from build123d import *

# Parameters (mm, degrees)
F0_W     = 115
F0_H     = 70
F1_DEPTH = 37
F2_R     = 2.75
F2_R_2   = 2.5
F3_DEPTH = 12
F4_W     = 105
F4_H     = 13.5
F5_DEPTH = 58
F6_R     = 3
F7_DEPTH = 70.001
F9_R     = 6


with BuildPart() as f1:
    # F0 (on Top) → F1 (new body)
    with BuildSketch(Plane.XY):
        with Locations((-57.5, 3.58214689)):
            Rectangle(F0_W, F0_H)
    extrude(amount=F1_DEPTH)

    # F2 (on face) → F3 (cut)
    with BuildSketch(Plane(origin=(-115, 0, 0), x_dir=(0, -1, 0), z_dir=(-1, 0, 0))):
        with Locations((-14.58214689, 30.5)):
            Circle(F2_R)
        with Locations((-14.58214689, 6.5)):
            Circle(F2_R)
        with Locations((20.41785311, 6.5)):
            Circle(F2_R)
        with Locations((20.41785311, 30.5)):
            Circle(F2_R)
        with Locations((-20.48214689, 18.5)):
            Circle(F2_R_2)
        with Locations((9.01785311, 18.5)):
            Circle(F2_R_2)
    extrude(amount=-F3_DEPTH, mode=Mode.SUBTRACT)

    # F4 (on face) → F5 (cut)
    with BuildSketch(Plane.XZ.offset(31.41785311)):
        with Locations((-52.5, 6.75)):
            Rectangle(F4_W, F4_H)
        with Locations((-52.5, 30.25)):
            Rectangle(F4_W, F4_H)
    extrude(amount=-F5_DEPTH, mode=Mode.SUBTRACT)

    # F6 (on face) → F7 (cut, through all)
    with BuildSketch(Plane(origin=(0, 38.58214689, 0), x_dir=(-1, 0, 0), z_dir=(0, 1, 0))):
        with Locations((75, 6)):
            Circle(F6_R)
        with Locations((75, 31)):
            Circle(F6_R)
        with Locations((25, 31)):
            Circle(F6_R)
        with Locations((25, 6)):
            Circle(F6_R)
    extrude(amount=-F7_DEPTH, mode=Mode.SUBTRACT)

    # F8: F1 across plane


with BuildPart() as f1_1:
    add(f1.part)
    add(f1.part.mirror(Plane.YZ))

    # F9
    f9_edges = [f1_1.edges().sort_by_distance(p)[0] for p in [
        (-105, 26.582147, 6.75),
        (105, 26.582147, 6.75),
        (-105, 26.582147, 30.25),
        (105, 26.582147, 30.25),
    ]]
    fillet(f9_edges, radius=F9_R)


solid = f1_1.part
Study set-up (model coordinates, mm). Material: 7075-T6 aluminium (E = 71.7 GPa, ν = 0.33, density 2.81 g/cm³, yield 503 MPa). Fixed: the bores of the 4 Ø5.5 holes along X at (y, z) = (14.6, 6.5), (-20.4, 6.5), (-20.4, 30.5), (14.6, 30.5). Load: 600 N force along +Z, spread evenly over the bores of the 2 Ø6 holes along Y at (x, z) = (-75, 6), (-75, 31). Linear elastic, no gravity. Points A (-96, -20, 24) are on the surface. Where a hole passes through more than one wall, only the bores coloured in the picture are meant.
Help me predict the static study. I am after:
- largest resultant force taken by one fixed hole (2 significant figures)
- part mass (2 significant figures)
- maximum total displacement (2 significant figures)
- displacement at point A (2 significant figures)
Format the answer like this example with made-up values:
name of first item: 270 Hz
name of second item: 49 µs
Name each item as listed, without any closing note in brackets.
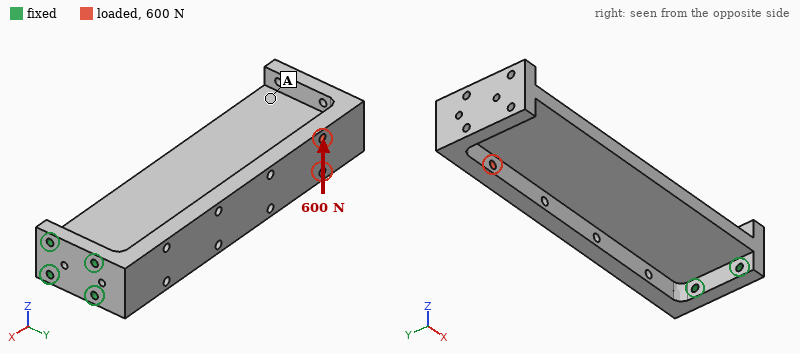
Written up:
largest resultant force taken by one fixed hole: 3.7 kN
part mass: 740 g
maximum total displacement: 0.74 mm
displacement at point A: 0.62 mm
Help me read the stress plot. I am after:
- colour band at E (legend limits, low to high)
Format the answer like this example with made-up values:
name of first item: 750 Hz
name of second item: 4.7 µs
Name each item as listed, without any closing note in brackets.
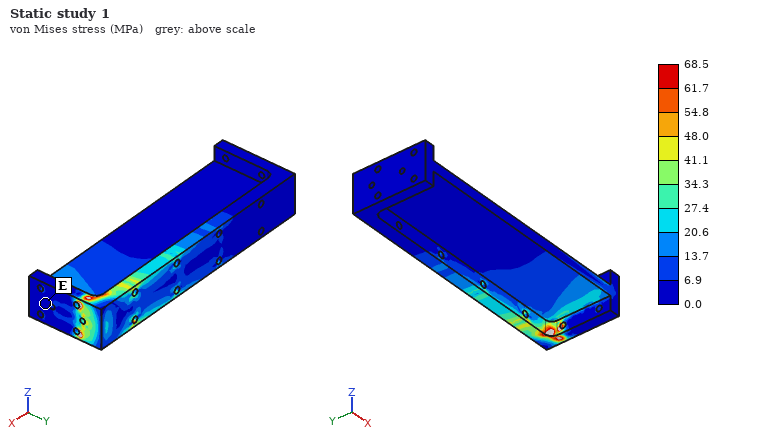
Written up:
colour band at E: 0.0 to 6.9 MPa
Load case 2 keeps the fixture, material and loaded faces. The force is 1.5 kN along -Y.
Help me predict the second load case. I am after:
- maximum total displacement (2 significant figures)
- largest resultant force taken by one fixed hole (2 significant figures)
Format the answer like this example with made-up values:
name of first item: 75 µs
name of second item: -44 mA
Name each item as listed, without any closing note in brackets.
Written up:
maximum total displacement: 0.26 mm
largest resultant force taken by one fixed hole: 3.4 kN
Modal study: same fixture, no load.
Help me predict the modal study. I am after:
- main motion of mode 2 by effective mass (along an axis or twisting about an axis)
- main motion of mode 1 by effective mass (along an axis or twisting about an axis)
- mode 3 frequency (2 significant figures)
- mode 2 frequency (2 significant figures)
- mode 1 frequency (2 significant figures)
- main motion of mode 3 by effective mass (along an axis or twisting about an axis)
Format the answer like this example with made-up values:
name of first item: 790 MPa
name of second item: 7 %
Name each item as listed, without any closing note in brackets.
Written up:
main motion of mode 2 by effective mass: along Y
main motion of mode 1 by effective mass: along Z
mode 3 frequency: 970 Hz
mode 2 frequency: 710 Hz
mode 1 frequency: 270 Hz
main motion of mode 3 by effective mass: twisting about X
